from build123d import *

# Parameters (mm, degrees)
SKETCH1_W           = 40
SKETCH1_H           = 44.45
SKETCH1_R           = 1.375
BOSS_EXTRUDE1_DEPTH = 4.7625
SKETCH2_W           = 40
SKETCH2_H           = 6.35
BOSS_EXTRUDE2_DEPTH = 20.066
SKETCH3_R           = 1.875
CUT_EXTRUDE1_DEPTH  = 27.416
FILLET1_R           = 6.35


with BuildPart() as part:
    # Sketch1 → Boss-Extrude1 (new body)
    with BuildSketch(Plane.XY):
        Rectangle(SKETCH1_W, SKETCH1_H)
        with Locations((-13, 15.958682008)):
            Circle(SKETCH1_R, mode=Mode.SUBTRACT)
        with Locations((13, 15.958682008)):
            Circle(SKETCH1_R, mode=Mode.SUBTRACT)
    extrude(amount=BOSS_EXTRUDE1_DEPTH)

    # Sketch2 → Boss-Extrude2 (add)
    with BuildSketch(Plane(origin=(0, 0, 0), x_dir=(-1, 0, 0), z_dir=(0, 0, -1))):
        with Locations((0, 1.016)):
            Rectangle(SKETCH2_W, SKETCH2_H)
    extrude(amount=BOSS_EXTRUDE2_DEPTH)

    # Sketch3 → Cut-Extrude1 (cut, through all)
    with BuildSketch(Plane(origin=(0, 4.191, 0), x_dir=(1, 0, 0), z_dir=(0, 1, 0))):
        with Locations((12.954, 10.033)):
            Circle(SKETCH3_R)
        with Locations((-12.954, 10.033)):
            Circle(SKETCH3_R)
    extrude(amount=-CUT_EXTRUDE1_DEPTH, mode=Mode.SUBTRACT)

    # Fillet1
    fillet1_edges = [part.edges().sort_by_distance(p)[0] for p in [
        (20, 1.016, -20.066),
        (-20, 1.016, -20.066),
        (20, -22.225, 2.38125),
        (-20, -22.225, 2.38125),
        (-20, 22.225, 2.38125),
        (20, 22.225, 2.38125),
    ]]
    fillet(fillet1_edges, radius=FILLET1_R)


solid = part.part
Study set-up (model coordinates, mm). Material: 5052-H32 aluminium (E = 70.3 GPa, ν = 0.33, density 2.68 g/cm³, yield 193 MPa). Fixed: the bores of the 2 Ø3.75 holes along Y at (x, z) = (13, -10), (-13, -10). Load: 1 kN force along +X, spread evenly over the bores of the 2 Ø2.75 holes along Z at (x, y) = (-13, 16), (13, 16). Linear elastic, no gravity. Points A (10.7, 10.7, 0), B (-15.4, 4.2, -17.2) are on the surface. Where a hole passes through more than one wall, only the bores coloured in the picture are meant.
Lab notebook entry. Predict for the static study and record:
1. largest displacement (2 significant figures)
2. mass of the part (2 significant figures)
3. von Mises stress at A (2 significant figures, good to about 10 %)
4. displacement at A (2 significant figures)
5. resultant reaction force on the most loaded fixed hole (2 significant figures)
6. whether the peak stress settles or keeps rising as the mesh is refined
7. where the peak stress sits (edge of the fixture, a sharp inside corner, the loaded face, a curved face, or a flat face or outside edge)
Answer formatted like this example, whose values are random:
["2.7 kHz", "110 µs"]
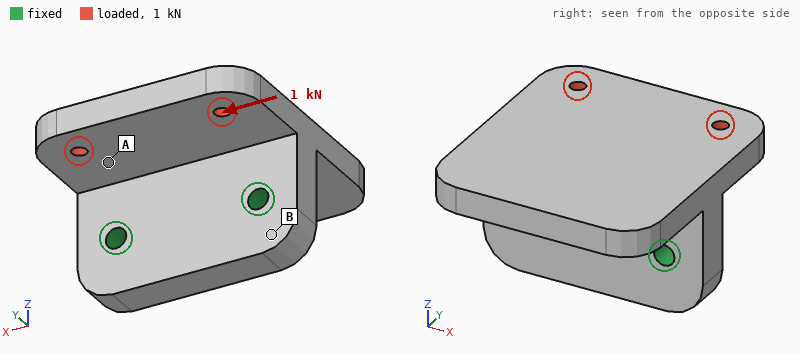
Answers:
["24 µm", "35 g", "17 MPa", "13 µm", "830 N", "keeps rising", "edge of the fixture"]
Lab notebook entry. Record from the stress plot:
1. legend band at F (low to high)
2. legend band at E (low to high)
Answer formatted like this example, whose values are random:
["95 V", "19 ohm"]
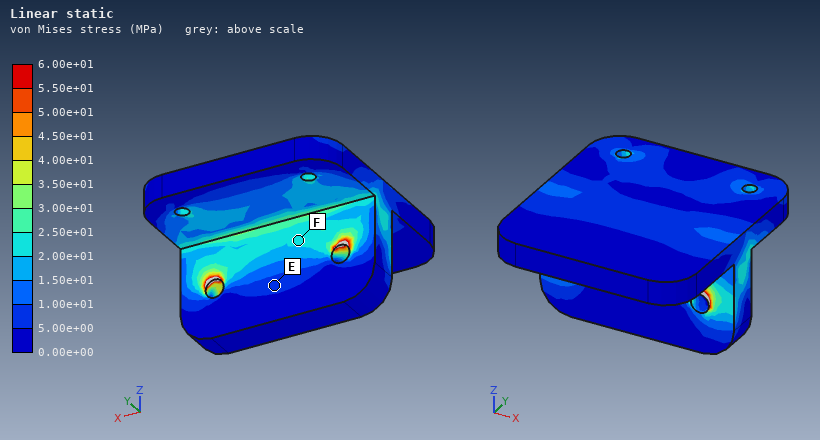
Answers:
["2.00e+01 to 2.50e+01 MPa", "5.00e+00 to 1.00e+01 MPa"]
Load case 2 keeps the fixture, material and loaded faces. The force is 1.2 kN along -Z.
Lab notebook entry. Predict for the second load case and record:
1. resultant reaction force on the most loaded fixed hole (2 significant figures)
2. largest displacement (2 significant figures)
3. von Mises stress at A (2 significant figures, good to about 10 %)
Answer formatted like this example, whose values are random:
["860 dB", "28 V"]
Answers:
["610 N", "0.15 mm", "40 MPa"]
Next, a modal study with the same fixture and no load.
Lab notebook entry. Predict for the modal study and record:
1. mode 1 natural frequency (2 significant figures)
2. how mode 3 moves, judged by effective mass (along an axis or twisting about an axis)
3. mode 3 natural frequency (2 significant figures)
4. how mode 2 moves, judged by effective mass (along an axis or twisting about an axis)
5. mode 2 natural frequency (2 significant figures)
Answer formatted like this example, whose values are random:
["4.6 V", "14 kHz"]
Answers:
["4600 Hz", "along Z", "9300 Hz", "twisting about Z", "8400 Hz"]
